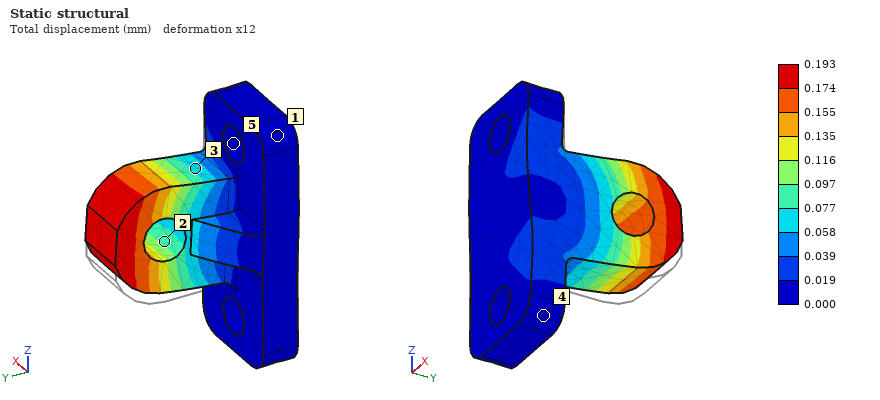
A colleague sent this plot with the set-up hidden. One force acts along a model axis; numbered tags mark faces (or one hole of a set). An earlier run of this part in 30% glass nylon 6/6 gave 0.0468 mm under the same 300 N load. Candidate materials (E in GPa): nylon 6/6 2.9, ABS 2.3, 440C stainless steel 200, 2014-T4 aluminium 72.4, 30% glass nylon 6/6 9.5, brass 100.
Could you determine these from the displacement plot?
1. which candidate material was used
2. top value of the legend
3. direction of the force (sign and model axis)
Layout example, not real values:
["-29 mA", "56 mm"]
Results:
["ABS", "0.193 mm", "+Z"]
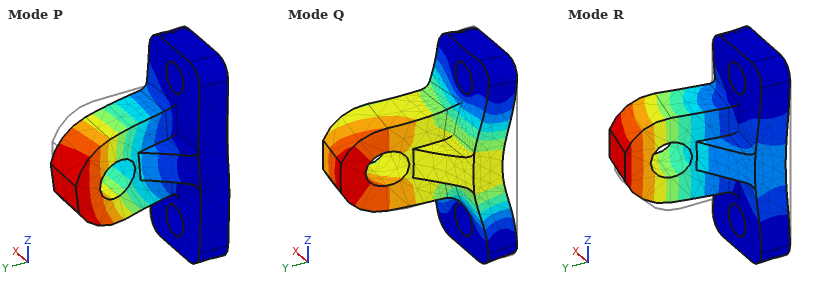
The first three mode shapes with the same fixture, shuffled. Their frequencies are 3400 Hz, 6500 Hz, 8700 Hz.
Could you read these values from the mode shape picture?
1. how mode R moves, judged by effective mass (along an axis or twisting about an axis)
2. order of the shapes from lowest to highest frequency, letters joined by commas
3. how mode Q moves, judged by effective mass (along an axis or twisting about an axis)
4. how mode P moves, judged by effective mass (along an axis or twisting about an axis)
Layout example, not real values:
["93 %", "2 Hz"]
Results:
["along X", "R, P, Q", "along Y", "along Z"]
